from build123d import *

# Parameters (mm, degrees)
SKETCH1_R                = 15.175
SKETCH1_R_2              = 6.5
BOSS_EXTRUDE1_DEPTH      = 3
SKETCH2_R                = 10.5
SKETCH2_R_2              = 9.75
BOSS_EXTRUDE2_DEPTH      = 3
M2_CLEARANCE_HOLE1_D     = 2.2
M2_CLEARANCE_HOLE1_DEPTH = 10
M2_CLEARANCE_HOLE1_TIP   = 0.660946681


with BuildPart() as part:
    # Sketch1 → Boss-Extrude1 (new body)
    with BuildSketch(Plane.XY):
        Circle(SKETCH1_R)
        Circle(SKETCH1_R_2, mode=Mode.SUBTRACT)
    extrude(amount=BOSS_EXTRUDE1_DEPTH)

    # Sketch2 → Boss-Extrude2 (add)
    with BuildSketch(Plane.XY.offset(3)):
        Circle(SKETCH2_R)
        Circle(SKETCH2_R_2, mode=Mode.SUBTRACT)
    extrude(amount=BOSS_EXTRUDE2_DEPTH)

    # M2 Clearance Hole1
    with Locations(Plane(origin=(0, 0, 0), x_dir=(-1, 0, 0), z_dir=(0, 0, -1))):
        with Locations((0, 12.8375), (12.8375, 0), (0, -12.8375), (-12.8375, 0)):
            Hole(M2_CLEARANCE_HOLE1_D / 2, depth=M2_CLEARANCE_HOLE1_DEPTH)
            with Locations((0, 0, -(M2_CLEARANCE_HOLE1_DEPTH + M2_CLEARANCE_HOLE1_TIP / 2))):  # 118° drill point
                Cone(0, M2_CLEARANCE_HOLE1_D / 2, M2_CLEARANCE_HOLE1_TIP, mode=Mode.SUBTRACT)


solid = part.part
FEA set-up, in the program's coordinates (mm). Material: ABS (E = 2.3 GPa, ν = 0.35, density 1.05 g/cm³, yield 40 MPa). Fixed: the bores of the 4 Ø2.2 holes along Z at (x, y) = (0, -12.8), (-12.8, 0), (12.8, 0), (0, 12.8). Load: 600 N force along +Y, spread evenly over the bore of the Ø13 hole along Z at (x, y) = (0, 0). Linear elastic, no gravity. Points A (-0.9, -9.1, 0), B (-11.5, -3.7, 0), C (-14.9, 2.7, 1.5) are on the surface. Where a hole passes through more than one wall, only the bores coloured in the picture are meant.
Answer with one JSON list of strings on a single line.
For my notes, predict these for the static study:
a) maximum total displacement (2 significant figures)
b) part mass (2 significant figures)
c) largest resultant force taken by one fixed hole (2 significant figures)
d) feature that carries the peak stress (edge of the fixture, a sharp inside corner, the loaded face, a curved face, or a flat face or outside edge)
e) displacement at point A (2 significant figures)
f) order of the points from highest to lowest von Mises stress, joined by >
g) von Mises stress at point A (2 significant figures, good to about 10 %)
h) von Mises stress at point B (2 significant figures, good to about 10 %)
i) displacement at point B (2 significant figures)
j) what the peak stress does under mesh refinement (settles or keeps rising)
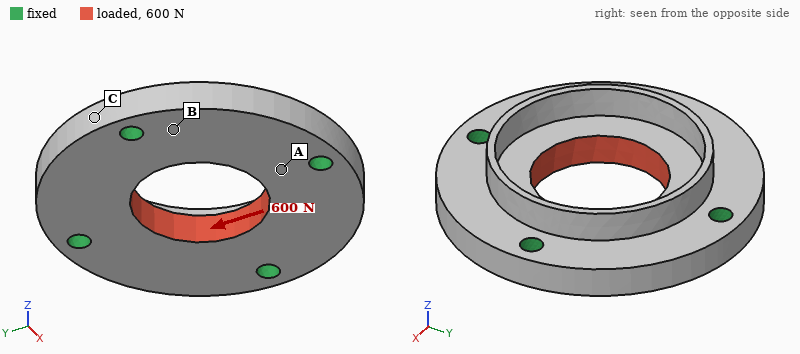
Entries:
["36 µm", "2.0 g", "170 N", "edge of the fixture", "13 µm", "A > B > C", "9.0 MPa", "4.9 MPa", "13 µm", "keeps rising"]
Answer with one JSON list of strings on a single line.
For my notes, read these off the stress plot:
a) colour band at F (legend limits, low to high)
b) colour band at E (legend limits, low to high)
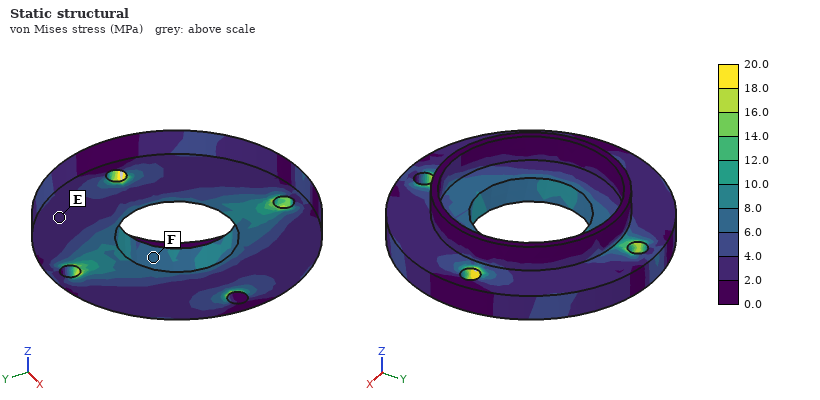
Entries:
["6.0 to 8.0 MPa", "2.0 to 4.0 MPa"]
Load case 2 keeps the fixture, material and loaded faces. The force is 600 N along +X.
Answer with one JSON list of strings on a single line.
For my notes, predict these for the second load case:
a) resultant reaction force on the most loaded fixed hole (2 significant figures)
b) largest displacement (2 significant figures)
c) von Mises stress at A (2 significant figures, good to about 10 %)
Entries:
["170 N", "36 µm", "3.1 MPa"]
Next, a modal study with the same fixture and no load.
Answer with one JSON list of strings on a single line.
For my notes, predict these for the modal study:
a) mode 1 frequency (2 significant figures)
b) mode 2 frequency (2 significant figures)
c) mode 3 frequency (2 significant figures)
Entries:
["9800 Hz", "11 kHz", "11 kHz"]
